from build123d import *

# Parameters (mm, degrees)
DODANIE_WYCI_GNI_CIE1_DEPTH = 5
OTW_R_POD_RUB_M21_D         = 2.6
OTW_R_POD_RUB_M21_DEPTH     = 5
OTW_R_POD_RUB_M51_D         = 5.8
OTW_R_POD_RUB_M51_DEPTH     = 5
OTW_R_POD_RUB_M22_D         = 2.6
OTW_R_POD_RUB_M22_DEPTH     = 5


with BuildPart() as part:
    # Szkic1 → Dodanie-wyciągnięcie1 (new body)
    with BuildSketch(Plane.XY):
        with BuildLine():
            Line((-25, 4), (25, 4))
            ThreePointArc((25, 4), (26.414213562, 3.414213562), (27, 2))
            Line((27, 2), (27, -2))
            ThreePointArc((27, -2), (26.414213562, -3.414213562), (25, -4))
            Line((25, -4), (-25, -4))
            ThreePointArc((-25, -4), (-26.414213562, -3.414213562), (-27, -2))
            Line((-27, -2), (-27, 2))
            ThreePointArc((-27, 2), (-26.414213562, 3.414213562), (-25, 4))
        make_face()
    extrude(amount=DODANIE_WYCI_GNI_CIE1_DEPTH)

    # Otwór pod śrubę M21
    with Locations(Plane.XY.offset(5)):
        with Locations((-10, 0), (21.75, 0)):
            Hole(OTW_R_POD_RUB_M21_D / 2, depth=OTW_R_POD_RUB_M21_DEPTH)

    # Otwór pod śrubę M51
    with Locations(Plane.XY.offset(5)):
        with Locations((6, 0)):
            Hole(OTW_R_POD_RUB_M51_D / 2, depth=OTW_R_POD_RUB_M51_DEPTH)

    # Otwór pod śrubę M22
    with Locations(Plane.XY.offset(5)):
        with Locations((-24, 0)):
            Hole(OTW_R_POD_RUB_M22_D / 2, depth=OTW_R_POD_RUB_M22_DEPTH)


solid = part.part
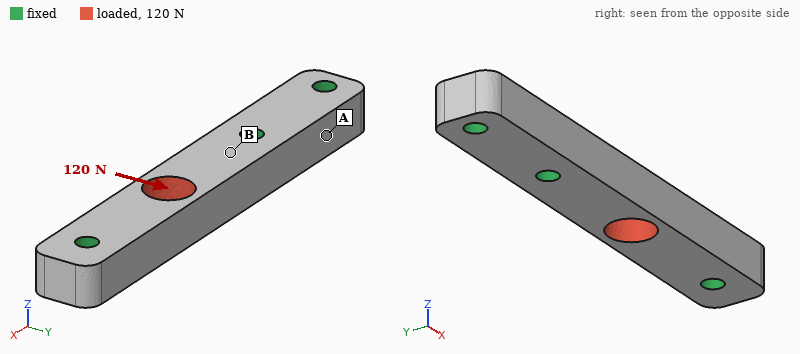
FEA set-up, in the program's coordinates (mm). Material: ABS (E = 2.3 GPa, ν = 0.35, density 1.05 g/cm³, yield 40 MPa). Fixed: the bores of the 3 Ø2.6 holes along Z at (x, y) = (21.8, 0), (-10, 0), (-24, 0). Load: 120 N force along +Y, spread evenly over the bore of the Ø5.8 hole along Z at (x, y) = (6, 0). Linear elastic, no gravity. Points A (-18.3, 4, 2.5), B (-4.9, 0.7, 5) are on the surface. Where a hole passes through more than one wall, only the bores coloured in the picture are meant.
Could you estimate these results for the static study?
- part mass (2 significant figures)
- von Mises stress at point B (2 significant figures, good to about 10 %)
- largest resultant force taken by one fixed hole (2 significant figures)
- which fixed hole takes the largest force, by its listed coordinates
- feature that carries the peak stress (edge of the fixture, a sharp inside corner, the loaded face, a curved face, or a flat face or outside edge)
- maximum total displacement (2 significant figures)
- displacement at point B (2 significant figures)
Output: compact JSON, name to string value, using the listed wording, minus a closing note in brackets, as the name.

{"part mass": "2.0 g", "von Mises stress at point B": "4.0 MPa", "largest resultant force taken by one fixed hole": "76 N", "which fixed hole takes the largest force, by its listed coordinates": "(-10, 0)", "feature that carries the peak stress": "edge of the fixture", "maximum total displacement": "94 µm", "displacement at point B": "27 µm"}
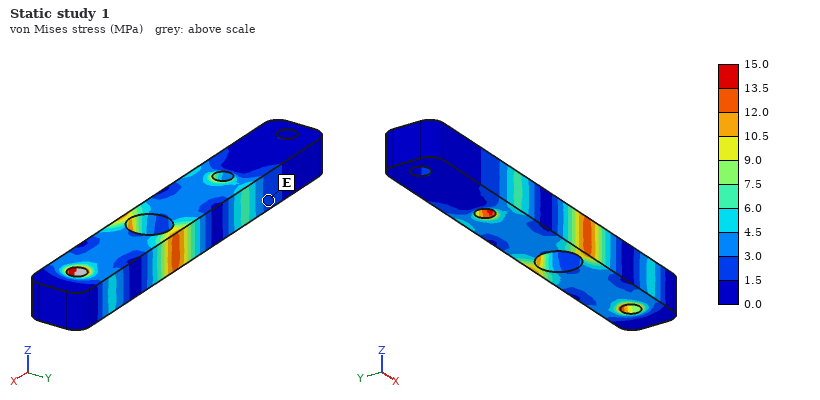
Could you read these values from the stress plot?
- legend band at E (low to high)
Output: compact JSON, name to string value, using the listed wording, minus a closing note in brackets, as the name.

{"legend band at E": "1.5 to 3.0 MPa"}
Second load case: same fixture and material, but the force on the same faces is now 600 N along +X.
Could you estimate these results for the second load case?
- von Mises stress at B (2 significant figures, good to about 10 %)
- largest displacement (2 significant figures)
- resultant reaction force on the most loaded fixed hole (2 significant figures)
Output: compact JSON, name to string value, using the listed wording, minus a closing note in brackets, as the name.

{"von Mises stress at B": "8.5 MPa", "largest displacement": "55 µm", "resultant reaction force on the most loaded fixed hole": "300 N"}
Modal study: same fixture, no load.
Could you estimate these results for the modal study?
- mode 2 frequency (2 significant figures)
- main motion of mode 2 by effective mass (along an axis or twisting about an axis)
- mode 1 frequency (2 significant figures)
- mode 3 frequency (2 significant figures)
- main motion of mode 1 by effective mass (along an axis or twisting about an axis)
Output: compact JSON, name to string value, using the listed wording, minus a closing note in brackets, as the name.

{"mode 2 frequency": "8500 Hz", "main motion of mode 2 by effective mass": "along Y", "mode 1 frequency": "6800 Hz", "mode 3 frequency": "12 kHz", "main motion of mode 1 by effective mass": "along Z"}
